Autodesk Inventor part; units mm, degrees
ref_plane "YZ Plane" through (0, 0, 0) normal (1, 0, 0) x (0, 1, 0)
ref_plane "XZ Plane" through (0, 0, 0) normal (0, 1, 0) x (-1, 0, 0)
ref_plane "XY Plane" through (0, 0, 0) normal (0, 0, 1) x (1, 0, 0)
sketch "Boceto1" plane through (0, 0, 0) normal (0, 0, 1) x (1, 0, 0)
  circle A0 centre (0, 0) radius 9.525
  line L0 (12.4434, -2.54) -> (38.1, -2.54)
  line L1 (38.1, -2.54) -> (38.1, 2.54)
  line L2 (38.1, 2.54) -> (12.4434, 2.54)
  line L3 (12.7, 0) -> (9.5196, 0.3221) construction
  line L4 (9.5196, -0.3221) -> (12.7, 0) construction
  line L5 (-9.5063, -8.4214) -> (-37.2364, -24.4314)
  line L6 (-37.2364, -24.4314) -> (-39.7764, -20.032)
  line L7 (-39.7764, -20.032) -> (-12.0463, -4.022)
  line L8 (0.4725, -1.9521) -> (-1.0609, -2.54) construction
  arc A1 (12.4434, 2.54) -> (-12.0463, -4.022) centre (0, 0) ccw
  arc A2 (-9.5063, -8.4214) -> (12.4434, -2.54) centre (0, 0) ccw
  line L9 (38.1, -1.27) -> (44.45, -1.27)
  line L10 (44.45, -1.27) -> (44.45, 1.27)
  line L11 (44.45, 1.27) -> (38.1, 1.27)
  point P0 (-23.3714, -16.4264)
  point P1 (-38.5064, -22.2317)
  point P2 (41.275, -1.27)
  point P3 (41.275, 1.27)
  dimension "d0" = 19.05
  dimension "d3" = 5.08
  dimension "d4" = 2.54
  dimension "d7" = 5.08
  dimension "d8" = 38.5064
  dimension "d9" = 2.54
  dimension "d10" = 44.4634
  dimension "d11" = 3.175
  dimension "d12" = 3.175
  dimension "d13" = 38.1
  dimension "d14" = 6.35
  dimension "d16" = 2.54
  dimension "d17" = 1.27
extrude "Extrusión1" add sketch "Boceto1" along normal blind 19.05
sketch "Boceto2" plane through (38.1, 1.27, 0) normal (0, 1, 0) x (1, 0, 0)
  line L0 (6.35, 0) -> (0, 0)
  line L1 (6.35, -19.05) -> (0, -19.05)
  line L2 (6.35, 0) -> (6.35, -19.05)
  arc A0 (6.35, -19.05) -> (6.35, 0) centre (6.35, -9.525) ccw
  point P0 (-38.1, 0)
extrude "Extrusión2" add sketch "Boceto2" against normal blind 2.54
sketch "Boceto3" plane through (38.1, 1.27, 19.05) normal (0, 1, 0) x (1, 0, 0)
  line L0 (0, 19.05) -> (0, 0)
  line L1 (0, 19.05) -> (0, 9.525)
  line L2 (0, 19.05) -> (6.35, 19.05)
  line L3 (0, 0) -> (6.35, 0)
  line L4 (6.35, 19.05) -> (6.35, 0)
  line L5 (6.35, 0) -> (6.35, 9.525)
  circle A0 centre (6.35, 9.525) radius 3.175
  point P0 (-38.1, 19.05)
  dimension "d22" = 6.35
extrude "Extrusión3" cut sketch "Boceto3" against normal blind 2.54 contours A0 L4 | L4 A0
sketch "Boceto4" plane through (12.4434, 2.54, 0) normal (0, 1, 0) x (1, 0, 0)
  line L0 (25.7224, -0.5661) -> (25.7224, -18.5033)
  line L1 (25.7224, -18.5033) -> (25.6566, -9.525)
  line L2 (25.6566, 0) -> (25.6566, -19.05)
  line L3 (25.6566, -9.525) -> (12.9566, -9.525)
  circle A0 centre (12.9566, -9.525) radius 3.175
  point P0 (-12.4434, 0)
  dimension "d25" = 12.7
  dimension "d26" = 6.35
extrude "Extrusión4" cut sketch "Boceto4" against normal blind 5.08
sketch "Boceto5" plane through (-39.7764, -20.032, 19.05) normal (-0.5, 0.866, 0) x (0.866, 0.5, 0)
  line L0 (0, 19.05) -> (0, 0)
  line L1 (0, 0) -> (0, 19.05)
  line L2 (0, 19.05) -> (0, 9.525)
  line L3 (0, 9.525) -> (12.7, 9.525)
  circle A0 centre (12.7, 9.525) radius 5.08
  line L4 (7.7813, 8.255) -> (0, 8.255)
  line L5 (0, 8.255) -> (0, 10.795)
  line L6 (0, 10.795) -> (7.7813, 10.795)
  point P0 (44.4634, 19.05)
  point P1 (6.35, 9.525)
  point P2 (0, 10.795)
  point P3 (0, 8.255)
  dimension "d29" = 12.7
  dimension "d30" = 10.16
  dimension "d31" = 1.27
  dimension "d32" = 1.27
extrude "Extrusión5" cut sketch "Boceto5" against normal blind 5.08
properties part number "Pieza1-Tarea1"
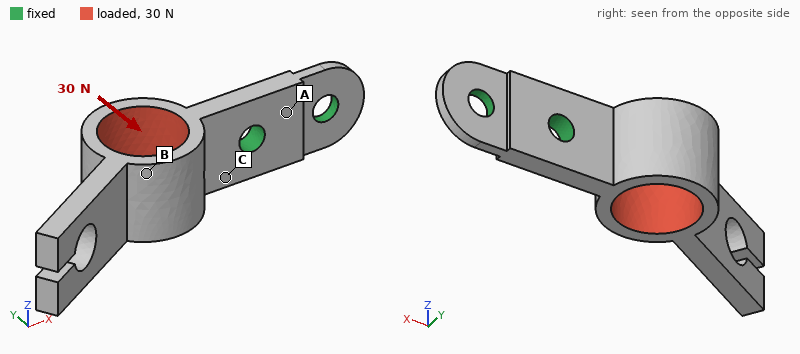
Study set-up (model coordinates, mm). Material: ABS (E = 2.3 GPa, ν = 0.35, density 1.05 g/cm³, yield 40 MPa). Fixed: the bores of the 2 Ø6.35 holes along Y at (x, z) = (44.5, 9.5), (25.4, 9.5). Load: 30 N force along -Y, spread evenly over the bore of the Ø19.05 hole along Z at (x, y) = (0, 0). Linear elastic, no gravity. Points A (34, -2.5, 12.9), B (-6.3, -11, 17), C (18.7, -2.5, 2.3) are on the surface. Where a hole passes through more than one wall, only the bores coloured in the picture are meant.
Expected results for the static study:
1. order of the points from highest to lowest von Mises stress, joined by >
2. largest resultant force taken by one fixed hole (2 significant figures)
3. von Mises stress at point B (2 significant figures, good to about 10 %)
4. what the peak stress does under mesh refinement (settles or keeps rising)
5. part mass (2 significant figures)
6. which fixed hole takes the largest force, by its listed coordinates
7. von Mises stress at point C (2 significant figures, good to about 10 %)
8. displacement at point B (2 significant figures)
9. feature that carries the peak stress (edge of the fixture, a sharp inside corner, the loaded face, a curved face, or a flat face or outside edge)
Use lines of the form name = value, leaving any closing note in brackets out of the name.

order of the points from highest to lowest von Mises stress, joined by > = C > B > A
largest resultant force taken by one fixed hole = 32 N
von Mises stress at point B = 1.3 MPa
what the peak stress does under mesh refinement = keeps rising
part mass = 10 g
which fixed hole takes the largest force, by its listed coordinates = (25.4, 9.5)
von Mises stress at point C = 5.6 MPa
displacement at point B = 0.50 mm
feature that carries the peak stress = edge of the fixture
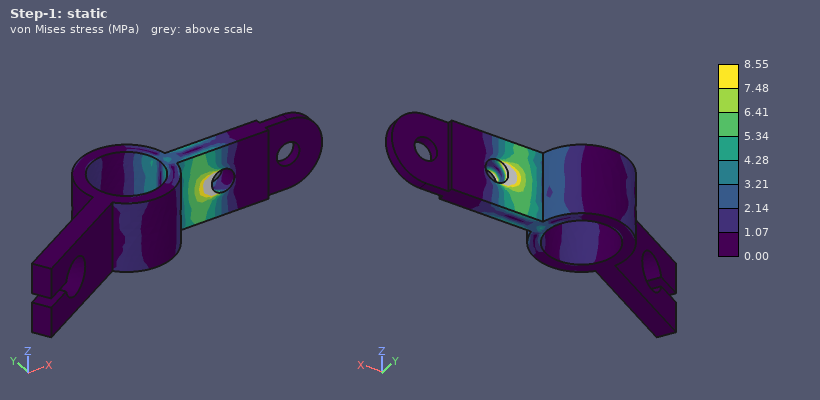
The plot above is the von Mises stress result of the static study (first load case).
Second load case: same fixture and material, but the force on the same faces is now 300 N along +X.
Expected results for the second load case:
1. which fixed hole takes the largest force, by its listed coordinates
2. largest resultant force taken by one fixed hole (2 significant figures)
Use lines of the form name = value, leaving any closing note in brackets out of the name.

which fixed hole takes the largest force, by its listed coordinates = (25.4, 9.5)
largest resultant force taken by one fixed hole = 280 N
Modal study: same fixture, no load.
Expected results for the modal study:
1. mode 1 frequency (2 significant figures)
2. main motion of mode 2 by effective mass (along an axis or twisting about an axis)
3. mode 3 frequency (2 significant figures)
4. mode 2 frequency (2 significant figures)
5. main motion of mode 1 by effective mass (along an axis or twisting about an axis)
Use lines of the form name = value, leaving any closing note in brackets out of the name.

mode 1 frequency = 300 Hz
main motion of mode 2 by effective mass = along Z
mode 3 frequency = 1400 Hz
mode 2 frequency = 550 Hz
main motion of mode 1 by effective mass = along Y
